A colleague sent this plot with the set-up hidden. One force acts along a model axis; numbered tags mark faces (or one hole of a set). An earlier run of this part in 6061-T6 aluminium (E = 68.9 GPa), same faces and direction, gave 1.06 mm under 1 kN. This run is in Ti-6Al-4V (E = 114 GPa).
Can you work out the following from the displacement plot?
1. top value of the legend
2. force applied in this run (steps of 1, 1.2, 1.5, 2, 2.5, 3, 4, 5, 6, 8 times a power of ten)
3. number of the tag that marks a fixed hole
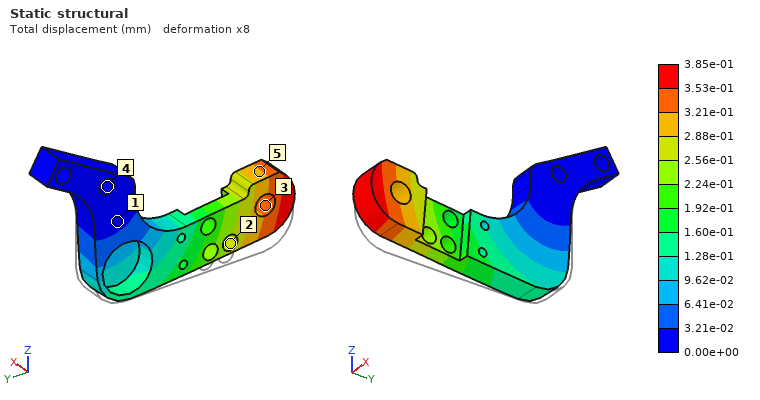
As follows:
3.85e-01 mm
600 N
4
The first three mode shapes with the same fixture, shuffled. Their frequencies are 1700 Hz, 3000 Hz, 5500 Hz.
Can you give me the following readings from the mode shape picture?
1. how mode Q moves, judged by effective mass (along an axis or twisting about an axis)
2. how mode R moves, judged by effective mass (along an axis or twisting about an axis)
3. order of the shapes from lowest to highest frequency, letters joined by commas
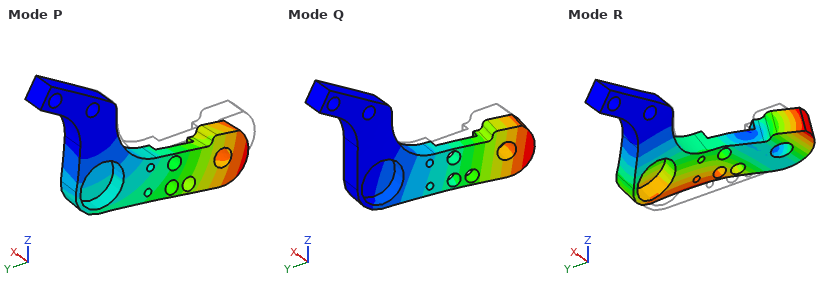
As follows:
along X
along X
Q, P, R
